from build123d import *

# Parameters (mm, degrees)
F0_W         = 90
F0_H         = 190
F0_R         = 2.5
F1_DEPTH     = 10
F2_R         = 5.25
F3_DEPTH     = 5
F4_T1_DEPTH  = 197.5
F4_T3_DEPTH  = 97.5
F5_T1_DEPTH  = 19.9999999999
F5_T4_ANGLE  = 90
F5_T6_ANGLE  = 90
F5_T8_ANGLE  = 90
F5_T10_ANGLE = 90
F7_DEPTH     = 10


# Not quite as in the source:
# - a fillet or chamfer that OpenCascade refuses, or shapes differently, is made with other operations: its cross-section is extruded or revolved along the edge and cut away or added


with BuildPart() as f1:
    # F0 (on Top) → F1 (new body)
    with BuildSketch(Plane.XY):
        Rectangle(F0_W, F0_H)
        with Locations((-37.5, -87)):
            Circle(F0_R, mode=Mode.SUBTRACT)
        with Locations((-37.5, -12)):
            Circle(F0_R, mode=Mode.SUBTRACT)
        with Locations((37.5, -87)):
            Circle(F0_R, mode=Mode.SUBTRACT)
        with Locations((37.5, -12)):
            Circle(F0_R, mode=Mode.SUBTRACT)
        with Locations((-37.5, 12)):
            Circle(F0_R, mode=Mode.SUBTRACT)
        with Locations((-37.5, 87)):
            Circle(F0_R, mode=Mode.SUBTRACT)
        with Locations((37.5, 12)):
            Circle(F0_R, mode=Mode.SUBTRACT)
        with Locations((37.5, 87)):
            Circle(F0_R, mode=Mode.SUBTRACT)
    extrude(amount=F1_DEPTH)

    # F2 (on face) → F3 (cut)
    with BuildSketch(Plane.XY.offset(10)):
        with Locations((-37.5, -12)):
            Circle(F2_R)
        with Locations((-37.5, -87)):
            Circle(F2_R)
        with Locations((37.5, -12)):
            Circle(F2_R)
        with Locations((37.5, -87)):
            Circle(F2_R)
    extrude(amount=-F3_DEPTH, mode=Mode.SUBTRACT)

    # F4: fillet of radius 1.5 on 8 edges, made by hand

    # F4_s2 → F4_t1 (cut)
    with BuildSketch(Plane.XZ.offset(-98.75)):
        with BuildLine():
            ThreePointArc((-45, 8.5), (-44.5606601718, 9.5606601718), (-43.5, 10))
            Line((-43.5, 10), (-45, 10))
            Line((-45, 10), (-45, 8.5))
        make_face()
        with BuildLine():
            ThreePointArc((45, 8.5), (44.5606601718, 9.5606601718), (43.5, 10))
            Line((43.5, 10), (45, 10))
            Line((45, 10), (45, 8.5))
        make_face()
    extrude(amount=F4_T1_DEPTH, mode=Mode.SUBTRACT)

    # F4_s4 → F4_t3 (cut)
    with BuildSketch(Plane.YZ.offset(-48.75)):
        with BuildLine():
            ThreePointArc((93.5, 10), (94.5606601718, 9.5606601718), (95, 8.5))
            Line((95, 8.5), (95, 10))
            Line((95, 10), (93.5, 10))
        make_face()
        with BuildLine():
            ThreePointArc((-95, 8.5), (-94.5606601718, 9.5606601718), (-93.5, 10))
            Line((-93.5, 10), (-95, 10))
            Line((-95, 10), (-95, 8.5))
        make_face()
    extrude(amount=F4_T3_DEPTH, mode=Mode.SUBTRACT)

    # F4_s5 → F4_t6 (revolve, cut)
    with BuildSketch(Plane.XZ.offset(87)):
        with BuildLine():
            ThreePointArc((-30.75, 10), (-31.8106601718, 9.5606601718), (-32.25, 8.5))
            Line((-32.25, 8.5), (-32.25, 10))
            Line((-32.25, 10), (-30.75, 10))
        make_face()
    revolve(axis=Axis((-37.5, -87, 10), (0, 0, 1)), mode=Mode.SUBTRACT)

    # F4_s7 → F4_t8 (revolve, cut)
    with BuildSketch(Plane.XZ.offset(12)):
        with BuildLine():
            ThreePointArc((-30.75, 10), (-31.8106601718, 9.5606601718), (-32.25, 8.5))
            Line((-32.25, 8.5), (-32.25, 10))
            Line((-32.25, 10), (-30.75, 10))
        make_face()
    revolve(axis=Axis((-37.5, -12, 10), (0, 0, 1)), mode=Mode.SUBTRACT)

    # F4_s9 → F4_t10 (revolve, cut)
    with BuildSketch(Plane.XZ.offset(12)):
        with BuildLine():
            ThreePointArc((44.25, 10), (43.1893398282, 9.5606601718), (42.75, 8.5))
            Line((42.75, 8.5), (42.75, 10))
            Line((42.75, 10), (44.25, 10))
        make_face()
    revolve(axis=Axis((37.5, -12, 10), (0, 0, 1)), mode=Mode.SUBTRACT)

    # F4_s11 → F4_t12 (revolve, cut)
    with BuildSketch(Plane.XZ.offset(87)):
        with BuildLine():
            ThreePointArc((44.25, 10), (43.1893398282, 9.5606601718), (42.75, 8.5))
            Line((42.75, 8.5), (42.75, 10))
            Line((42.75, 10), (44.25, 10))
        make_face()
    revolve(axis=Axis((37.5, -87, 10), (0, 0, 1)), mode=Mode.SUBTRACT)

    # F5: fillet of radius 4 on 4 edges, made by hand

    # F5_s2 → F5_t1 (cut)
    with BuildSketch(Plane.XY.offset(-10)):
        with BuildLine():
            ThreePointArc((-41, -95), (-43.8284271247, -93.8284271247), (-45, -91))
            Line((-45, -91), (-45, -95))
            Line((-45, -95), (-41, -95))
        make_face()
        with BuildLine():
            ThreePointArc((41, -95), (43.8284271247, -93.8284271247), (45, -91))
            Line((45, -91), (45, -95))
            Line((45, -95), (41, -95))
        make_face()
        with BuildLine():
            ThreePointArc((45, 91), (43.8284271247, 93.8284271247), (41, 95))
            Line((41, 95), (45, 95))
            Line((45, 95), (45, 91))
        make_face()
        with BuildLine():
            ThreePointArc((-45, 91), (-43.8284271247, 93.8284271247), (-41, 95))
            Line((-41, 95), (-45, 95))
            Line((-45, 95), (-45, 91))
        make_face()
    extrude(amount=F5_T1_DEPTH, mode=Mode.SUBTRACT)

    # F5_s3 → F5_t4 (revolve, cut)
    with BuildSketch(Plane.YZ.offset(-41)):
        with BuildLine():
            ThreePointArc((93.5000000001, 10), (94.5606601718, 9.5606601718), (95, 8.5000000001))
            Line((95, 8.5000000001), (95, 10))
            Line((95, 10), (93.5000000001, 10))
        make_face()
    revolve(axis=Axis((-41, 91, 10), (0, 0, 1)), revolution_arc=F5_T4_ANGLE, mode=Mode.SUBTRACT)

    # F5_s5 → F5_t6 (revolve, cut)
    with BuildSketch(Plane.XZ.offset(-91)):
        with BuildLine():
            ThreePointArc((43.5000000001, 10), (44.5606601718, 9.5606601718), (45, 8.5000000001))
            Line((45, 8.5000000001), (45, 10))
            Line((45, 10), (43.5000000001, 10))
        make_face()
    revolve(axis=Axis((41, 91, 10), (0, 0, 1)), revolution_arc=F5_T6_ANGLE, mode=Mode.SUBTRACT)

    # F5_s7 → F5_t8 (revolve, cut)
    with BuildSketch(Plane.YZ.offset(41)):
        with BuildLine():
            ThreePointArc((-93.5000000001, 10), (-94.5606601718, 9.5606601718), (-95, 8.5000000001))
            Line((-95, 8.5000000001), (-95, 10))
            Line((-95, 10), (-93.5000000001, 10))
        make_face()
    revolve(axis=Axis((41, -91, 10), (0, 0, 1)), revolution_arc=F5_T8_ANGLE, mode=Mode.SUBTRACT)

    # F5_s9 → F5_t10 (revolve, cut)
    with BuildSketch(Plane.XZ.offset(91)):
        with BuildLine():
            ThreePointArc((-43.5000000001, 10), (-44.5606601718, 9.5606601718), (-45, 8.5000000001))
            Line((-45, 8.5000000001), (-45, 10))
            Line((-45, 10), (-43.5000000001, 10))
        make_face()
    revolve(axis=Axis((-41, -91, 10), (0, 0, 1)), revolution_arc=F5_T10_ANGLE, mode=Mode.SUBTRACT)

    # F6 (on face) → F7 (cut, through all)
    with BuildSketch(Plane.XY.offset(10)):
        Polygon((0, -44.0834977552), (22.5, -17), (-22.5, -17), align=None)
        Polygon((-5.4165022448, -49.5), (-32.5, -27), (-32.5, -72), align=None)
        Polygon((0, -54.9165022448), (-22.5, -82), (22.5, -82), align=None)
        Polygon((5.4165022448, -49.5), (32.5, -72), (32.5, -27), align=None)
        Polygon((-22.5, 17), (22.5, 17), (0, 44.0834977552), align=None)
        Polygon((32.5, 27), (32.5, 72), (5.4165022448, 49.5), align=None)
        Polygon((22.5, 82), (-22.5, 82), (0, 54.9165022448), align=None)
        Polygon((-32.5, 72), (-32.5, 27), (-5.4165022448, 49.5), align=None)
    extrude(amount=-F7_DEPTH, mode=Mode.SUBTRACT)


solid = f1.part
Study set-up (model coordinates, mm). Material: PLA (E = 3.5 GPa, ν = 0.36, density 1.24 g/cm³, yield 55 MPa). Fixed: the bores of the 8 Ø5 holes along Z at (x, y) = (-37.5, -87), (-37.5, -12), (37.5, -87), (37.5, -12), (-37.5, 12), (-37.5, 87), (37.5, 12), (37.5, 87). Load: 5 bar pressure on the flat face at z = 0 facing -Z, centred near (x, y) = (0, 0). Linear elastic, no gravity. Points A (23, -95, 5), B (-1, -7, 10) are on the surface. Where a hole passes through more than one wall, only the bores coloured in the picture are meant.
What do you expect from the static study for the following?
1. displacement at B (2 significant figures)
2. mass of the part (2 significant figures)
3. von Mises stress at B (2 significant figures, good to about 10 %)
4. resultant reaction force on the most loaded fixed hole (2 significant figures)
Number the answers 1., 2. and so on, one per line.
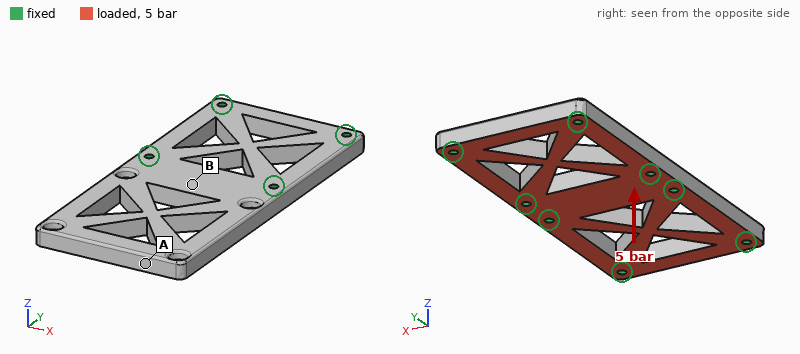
1. 0.27 mm
2. 150 g
3. 10.0 MPa
4. 990 N
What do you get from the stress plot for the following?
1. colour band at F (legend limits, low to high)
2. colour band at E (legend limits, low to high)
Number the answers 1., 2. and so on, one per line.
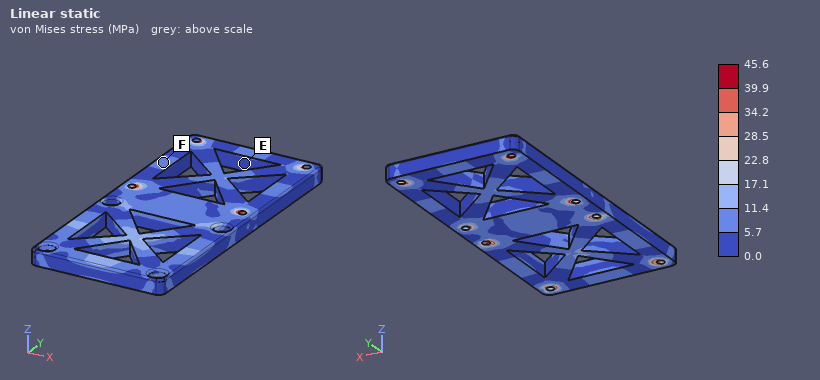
1. 5.7 to 11.4 MPa
2. 0.0 to 5.7 MPa
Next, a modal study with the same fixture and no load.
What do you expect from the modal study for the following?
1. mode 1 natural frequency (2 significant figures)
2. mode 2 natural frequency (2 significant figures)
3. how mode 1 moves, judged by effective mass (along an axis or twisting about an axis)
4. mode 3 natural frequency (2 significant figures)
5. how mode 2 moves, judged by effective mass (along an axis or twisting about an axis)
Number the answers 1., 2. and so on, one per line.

1. 1600 Hz
2. 1900 Hz
3. along Z
4. 2400 Hz
5. along Z
